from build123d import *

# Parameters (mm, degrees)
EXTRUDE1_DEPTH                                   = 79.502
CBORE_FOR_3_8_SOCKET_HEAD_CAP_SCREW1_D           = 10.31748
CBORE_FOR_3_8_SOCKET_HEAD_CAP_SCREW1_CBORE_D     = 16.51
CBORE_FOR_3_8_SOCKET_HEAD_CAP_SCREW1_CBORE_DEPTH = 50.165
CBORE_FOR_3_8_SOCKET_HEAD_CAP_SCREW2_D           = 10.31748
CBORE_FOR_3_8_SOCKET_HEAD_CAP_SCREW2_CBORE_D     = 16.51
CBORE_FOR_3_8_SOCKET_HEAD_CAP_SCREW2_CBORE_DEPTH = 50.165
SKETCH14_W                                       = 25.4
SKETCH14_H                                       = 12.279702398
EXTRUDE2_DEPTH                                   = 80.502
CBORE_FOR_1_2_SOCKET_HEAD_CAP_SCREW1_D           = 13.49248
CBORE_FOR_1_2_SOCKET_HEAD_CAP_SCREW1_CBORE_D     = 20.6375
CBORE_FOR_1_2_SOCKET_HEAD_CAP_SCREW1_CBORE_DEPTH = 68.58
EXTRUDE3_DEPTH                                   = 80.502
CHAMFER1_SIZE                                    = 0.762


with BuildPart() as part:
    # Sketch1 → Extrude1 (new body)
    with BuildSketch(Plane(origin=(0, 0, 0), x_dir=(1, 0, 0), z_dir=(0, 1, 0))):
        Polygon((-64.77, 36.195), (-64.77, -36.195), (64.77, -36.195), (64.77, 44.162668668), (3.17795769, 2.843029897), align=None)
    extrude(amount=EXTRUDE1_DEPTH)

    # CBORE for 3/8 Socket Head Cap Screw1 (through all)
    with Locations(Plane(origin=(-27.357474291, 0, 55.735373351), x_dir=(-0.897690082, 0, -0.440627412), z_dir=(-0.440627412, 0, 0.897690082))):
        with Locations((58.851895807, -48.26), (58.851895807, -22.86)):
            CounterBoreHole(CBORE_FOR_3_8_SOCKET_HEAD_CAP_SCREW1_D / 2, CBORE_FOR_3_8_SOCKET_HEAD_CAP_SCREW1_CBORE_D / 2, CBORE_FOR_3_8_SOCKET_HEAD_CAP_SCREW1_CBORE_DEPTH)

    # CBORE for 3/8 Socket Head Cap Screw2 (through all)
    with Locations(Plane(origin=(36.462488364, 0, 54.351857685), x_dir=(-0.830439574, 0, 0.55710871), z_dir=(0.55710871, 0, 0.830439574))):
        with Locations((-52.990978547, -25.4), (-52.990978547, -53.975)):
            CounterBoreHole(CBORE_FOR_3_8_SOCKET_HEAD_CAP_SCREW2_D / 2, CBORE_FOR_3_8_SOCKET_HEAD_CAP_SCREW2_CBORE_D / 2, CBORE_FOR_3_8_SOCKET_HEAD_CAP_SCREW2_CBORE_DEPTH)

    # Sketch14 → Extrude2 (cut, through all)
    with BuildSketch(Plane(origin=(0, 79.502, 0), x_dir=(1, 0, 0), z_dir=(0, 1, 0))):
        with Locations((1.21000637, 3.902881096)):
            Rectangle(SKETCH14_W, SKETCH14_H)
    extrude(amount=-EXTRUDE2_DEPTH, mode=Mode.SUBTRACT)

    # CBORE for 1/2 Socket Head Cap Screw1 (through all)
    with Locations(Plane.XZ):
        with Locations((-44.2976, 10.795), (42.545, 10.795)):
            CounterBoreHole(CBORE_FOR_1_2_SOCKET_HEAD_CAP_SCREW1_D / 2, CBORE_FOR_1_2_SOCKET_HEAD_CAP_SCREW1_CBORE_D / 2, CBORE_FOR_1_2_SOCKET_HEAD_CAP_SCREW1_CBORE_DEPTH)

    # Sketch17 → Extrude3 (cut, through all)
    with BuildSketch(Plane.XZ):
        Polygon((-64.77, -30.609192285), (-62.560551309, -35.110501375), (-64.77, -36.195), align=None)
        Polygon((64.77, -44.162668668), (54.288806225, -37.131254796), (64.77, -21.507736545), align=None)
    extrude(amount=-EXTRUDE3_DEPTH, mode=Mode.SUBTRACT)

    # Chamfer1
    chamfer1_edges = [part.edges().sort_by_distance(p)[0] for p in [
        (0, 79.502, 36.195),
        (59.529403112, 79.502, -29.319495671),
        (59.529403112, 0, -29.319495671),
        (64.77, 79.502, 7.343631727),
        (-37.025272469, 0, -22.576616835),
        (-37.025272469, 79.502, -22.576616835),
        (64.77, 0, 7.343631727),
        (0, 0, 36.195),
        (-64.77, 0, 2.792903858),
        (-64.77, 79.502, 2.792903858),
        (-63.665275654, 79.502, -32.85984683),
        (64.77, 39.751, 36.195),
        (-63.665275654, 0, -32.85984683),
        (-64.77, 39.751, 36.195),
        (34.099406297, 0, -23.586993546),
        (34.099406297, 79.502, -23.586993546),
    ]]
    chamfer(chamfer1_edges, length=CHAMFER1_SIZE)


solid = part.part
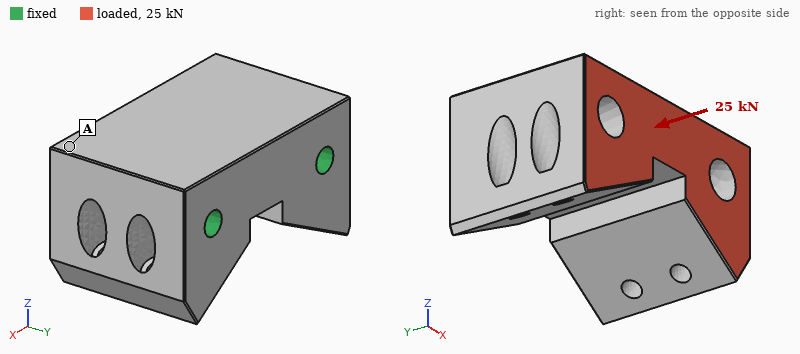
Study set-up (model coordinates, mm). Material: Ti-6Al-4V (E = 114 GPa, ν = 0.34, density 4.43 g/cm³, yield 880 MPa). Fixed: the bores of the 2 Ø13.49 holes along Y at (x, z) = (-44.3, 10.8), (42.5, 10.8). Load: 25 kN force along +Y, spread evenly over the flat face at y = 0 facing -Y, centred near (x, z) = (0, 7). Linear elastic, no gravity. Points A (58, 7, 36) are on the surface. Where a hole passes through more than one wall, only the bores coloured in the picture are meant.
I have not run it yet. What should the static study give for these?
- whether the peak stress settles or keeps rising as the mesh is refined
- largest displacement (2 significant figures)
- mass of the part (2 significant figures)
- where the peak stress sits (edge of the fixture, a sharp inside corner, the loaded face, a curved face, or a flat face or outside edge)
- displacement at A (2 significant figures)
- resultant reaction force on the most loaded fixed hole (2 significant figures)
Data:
keeps rising
27 µm
2.2 kg
edge of the fixture
16 µm
13 kN
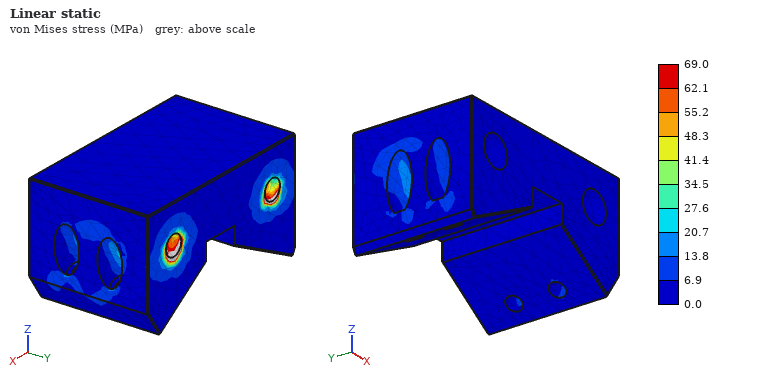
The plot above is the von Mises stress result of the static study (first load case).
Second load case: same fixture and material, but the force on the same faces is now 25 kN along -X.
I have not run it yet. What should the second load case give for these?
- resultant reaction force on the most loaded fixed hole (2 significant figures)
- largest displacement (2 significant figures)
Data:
24 kN
49 µm
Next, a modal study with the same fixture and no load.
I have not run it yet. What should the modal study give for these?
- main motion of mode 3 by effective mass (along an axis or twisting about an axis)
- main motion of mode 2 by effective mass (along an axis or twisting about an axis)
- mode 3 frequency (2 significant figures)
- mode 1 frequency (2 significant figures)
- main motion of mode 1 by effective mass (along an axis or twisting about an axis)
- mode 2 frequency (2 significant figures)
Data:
along X
along X
4700 Hz
1500 Hz
along Z
4000 Hz
